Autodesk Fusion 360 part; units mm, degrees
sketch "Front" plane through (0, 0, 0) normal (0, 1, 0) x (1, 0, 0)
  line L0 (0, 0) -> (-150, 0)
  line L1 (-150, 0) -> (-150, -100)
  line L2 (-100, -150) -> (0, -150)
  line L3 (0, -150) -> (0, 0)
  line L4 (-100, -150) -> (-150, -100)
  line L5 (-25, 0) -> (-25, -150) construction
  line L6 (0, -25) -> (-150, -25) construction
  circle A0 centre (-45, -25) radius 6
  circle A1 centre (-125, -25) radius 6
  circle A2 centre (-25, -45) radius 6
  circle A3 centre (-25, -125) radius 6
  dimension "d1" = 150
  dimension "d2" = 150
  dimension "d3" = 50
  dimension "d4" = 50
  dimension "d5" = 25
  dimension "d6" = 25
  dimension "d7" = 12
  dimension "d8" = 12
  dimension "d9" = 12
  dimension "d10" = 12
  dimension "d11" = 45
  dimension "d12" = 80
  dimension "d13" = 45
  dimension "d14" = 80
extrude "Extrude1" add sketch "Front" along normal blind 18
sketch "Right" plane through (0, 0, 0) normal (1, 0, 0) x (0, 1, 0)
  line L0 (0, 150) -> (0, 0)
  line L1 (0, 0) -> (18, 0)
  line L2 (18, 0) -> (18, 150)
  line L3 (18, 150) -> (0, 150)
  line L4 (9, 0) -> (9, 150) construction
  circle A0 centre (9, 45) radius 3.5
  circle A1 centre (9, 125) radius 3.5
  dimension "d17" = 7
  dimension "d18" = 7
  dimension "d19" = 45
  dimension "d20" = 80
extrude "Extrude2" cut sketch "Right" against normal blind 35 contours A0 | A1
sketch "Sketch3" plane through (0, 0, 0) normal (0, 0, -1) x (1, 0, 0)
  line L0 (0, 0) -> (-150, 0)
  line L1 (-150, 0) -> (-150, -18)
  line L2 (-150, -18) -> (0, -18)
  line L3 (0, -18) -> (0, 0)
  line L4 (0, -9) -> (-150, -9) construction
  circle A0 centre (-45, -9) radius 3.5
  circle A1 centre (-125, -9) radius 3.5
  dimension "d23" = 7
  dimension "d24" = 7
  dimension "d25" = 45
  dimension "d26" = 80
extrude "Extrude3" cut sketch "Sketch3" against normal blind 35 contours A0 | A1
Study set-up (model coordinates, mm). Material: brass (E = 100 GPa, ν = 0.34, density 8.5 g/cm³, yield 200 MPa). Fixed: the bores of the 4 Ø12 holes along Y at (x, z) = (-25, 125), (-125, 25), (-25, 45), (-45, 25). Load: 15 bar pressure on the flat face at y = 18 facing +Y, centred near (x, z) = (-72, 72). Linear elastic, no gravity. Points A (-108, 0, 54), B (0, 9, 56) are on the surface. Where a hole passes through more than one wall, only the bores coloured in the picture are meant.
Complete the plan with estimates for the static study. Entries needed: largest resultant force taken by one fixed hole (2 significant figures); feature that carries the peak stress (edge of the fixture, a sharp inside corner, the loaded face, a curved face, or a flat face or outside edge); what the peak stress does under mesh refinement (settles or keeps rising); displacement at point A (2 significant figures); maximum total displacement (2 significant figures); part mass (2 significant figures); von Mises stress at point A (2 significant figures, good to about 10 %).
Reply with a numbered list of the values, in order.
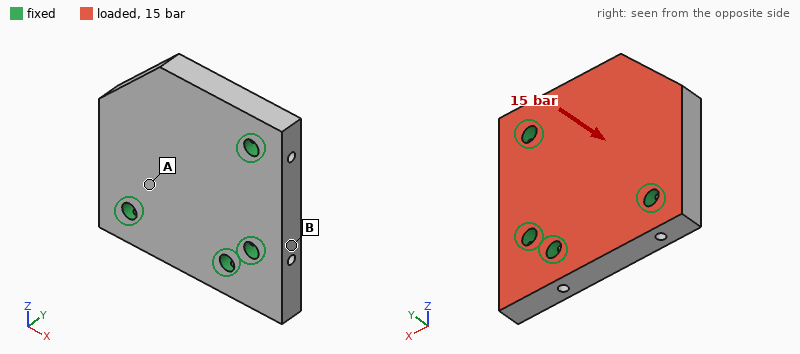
1. 11 kN
2. edge of the fixture
3. keeps rising
4. 0.037 mm
5. 0.17 mm
6. 3.2 kg
7. 27 MPa
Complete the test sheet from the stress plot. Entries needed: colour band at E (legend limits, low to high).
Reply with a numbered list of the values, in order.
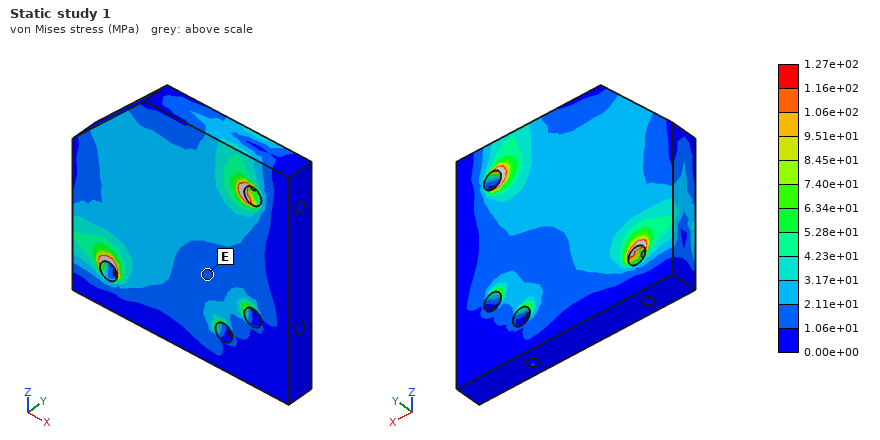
1. 1.06e+01 to 2.11e+01 MPa
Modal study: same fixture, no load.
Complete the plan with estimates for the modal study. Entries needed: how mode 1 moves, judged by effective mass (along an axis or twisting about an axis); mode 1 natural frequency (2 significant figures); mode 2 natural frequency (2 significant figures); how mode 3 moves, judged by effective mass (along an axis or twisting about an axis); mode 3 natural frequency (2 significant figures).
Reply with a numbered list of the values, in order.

1. along Y
2. 1600 Hz
3. 4000 Hz
4. along Y
5. 5000 Hz
